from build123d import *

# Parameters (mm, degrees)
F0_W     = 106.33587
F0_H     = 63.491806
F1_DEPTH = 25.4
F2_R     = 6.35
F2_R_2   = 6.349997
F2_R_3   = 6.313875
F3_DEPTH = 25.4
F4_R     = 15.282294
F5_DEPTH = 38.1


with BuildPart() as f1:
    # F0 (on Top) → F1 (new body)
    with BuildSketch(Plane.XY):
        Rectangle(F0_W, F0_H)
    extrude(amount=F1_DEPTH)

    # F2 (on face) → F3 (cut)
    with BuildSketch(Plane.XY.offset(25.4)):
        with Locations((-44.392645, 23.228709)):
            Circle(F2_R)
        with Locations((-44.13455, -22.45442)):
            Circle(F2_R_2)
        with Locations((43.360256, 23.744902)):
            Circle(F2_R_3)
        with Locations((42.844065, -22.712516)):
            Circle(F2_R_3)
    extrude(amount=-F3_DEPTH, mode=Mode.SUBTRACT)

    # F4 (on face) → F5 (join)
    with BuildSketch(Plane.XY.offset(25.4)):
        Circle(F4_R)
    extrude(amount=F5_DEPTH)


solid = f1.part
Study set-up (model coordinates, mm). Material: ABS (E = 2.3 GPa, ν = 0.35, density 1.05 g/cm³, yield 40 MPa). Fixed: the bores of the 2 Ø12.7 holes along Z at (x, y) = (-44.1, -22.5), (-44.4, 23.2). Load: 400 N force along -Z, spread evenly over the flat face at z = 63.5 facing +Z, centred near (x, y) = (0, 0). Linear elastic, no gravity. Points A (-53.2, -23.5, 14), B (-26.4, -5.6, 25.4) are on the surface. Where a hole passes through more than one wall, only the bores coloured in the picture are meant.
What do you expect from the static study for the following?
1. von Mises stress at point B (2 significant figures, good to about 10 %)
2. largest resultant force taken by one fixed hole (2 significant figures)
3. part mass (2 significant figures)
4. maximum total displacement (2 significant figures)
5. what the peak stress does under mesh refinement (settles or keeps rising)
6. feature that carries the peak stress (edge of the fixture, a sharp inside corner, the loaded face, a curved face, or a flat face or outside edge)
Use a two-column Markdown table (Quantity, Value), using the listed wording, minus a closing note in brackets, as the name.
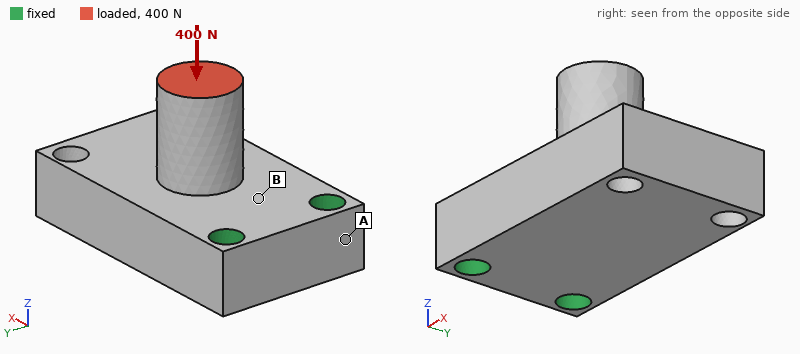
| Quantity | Value |
|---|---|
| von Mises stress at point B | 1.2 MPa |
| largest resultant force taken by one fixed hole | 200 N |
| part mass | 200 g |
| maximum total displacement | 0.18 mm |
| what the peak stress does under mesh refinement | keeps rising |
| feature that carries the peak stress | edge of the fixture |
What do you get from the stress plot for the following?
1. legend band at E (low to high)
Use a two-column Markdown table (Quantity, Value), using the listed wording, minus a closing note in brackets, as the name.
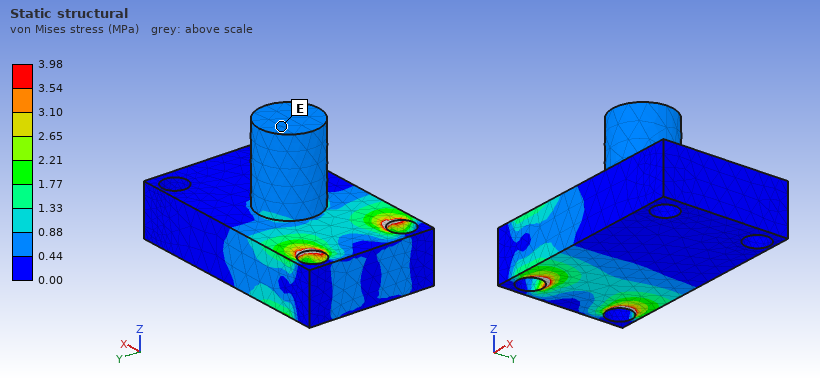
| Quantity | Value |
|---|---|
| legend band at E | 0.44 to 0.88 MPa |
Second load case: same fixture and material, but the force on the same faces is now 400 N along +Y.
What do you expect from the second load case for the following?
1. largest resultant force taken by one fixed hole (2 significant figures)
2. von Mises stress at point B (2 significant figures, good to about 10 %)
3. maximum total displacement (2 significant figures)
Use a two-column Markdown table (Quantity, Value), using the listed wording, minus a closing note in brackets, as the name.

| Quantity | Value |
|---|---|
| largest resultant force taken by one fixed hole | 540 N |
| von Mises stress at point B | 2.3 MPa |
| maximum total displacement | 0.28 mm |
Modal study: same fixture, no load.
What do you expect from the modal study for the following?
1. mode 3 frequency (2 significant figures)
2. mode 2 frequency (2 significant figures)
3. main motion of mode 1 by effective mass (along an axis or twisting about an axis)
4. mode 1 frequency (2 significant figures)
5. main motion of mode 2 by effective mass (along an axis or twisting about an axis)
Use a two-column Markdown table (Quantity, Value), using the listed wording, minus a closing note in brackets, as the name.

| Quantity | Value |
|---|---|
| mode 3 frequency | 1500 Hz |
| mode 2 frequency | 1300 Hz |
| main motion of mode 1 by effective mass | along Z |
| mode 1 frequency | 610 Hz |
| main motion of mode 2 by effective mass | along Y |
